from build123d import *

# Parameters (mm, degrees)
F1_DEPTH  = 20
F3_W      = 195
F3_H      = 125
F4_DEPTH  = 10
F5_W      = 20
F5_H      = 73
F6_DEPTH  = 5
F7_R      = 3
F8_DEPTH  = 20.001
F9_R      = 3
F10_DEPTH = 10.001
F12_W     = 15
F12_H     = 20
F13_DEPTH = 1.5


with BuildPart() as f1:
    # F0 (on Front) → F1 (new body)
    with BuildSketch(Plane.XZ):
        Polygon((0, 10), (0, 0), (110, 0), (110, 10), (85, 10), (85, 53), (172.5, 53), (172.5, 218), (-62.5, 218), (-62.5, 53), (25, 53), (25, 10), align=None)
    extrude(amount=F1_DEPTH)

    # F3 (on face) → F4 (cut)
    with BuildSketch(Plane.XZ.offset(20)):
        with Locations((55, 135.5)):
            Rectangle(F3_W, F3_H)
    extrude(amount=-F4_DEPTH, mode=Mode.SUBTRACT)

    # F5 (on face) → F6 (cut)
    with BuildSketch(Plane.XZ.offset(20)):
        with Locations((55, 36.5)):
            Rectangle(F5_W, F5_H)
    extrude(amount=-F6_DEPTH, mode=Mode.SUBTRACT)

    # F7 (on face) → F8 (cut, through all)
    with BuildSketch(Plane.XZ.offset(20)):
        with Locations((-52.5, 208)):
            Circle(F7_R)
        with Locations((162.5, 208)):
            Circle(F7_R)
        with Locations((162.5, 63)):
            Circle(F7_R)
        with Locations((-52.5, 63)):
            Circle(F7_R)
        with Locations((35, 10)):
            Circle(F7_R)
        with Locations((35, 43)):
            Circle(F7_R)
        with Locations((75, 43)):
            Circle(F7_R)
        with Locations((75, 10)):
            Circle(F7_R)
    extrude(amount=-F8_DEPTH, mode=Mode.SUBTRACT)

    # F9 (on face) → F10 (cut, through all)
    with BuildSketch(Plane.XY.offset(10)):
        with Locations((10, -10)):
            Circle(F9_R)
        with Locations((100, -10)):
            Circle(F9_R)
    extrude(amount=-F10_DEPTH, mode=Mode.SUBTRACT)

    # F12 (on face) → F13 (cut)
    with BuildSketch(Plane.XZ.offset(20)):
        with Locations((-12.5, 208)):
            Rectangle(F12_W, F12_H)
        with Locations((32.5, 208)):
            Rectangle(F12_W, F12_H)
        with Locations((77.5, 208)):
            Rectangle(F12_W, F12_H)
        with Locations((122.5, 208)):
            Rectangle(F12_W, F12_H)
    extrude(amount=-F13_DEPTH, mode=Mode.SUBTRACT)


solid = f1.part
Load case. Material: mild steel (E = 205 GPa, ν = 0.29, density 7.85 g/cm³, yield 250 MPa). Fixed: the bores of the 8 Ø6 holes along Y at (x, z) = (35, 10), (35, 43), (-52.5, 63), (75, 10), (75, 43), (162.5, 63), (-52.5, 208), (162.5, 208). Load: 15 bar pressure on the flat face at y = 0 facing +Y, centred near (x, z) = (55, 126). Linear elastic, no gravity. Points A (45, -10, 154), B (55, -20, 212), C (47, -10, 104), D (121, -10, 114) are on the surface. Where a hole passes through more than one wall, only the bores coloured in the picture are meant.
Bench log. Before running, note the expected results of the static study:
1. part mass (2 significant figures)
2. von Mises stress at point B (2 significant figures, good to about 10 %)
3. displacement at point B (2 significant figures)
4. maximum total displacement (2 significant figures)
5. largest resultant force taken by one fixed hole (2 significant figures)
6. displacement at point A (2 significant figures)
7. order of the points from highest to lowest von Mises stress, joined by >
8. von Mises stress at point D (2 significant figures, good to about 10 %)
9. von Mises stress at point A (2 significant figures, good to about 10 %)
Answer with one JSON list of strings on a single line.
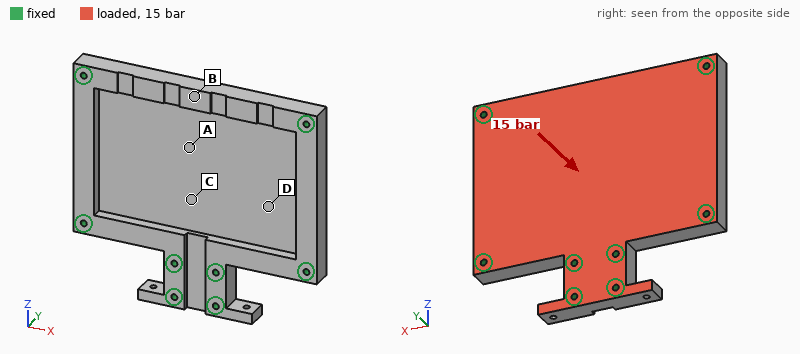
["4.6 kg", "100 MPa", "0.16 mm", "0.22 mm", "18 kN", "0.21 mm", "B > A > D > C", "43 MPa", "70 MPa"]
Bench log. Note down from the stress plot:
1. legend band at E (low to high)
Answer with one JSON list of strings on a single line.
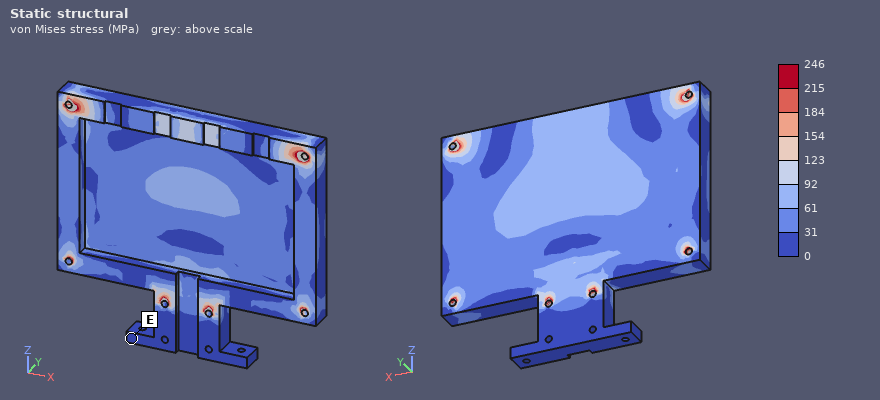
["0 to 31 MPa"]
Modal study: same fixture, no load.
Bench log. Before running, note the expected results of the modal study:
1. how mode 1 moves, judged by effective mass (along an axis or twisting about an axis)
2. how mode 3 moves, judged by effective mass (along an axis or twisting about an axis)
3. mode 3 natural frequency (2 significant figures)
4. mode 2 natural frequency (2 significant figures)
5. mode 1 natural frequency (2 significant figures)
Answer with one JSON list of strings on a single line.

["along Y", "twisting about Z", "3200 Hz", "2800 Hz", "1700 Hz"]
